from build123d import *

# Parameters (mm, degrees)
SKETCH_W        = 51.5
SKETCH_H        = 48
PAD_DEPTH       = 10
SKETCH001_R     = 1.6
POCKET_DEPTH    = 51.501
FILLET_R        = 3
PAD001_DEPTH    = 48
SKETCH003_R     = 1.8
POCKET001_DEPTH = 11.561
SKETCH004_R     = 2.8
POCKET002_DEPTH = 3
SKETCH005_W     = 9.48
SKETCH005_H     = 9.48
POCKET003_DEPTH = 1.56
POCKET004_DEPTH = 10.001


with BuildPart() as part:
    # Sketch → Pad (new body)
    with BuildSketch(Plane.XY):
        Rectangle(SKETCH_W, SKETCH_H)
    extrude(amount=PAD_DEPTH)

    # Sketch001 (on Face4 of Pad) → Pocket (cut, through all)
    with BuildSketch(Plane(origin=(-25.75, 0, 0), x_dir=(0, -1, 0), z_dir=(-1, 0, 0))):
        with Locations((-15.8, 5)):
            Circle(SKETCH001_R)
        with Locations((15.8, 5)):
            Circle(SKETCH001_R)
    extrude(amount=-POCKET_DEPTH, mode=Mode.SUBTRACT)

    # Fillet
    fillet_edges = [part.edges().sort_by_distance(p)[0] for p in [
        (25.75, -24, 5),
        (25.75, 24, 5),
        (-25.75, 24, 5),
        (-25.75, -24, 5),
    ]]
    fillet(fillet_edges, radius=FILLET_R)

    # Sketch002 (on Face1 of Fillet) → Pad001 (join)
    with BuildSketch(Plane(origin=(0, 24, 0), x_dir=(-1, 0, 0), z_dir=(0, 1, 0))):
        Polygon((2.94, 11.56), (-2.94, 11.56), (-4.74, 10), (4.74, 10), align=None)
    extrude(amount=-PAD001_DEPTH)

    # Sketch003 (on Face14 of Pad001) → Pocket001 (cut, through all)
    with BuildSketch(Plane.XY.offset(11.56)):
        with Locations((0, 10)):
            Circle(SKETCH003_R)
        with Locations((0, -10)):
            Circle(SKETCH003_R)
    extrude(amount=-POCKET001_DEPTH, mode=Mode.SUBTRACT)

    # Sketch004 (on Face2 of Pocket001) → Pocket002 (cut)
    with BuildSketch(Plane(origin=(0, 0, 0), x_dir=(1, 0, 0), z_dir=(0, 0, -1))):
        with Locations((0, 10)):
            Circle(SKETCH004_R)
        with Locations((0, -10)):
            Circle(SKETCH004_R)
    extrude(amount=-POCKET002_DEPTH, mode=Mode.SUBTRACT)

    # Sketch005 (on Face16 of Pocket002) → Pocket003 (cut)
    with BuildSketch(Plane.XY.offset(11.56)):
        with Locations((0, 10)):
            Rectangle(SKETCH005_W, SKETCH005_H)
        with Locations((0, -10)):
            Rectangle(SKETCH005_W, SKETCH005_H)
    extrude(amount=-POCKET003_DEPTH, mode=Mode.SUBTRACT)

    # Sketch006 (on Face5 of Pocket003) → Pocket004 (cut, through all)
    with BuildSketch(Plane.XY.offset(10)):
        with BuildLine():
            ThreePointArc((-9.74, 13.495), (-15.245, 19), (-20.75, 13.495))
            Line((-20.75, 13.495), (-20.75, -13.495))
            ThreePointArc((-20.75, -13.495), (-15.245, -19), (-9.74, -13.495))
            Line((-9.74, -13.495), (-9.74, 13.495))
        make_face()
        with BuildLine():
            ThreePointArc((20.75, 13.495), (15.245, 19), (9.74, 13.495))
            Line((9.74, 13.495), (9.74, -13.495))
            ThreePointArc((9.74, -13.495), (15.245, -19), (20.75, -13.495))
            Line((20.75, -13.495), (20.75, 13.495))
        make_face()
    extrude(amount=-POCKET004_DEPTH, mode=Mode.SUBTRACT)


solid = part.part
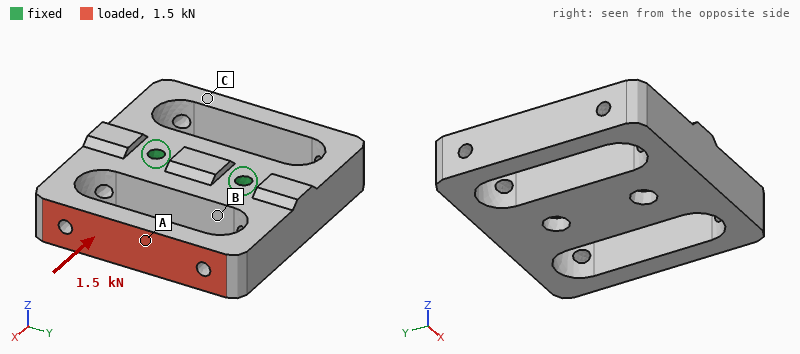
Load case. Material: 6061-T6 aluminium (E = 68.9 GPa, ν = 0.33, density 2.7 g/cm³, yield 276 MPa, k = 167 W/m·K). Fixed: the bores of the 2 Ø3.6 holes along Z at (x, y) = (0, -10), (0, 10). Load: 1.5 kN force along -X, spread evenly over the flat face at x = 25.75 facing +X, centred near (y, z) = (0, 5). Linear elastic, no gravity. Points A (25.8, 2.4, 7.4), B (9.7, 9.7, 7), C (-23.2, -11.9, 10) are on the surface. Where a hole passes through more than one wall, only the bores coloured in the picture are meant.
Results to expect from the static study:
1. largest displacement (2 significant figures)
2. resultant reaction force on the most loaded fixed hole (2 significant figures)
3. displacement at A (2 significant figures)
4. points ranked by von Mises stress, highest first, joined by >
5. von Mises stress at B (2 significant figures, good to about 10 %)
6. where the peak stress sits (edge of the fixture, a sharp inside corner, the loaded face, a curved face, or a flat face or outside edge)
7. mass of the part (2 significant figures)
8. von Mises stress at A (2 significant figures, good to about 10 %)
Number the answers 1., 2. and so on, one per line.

1. 64 µm
2. 770 N
3. 61 µm
4. A > B > C
5. 20 MPa
6. a curved face
7. 44 g
8. 73 MPa
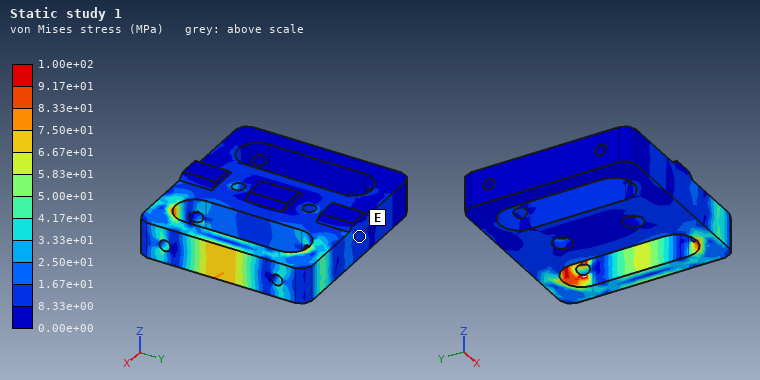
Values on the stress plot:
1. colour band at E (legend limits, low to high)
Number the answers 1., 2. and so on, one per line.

1. 8.33e+00 to 1.67e+01 MPa
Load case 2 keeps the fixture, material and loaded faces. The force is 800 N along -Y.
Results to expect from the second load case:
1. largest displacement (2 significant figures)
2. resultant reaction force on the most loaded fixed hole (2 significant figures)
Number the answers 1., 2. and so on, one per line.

1. 39 µm
2. 940 N
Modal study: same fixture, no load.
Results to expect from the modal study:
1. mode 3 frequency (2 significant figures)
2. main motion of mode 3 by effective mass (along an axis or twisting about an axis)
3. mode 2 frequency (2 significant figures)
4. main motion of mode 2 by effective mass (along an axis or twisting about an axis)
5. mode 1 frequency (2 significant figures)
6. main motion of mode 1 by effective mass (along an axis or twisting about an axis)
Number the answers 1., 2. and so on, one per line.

1. 7900 Hz
2. twisting about Z
3. 7300 Hz
4. along Z
5. 5200 Hz
6. twisting about Y
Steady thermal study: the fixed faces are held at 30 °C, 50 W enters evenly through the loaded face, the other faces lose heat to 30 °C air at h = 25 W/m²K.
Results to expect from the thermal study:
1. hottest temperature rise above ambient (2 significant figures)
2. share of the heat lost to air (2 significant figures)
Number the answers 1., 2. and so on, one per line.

1. 80 K
2. 6.2 %
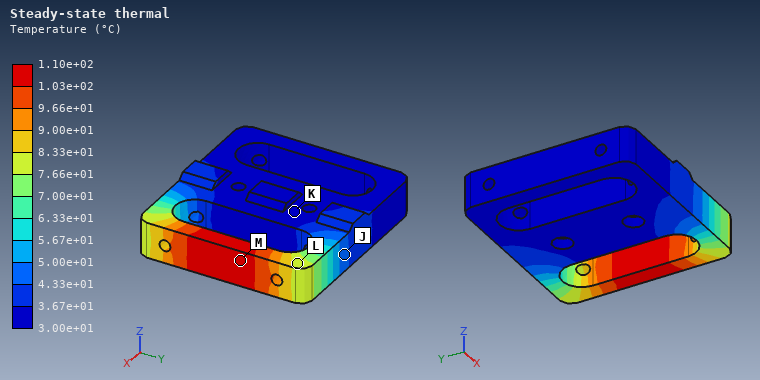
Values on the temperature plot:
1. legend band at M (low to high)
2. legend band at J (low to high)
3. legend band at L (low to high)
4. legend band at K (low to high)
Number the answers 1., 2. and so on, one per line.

1. 1.03e+02 to 1.10e+02 °C
2. 4.33e+01 to 5.00e+01 °C
3. 7.66e+01 to 8.33e+01 °C
4. 3.00e+01 to 3.67e+01 °C
